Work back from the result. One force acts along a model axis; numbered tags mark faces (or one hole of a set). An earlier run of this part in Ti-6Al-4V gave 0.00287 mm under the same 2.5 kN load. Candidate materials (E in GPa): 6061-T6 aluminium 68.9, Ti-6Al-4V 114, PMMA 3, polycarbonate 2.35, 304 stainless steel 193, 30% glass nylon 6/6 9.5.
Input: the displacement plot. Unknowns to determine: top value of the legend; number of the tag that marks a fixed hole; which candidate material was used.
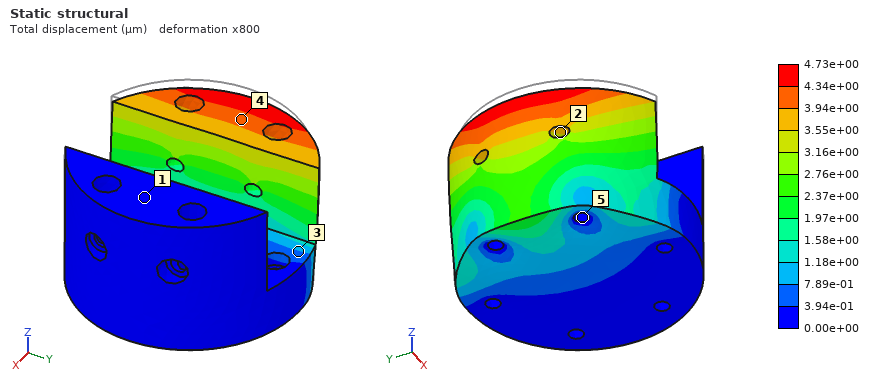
4.73e+00 µm
5
6061-T6 aluminium
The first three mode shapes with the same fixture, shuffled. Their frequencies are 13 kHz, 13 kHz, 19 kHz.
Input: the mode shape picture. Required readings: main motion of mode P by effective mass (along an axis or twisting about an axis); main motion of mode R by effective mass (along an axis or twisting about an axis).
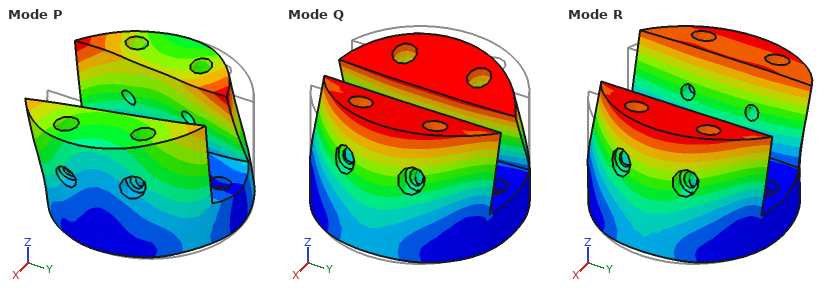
along Y
along X
